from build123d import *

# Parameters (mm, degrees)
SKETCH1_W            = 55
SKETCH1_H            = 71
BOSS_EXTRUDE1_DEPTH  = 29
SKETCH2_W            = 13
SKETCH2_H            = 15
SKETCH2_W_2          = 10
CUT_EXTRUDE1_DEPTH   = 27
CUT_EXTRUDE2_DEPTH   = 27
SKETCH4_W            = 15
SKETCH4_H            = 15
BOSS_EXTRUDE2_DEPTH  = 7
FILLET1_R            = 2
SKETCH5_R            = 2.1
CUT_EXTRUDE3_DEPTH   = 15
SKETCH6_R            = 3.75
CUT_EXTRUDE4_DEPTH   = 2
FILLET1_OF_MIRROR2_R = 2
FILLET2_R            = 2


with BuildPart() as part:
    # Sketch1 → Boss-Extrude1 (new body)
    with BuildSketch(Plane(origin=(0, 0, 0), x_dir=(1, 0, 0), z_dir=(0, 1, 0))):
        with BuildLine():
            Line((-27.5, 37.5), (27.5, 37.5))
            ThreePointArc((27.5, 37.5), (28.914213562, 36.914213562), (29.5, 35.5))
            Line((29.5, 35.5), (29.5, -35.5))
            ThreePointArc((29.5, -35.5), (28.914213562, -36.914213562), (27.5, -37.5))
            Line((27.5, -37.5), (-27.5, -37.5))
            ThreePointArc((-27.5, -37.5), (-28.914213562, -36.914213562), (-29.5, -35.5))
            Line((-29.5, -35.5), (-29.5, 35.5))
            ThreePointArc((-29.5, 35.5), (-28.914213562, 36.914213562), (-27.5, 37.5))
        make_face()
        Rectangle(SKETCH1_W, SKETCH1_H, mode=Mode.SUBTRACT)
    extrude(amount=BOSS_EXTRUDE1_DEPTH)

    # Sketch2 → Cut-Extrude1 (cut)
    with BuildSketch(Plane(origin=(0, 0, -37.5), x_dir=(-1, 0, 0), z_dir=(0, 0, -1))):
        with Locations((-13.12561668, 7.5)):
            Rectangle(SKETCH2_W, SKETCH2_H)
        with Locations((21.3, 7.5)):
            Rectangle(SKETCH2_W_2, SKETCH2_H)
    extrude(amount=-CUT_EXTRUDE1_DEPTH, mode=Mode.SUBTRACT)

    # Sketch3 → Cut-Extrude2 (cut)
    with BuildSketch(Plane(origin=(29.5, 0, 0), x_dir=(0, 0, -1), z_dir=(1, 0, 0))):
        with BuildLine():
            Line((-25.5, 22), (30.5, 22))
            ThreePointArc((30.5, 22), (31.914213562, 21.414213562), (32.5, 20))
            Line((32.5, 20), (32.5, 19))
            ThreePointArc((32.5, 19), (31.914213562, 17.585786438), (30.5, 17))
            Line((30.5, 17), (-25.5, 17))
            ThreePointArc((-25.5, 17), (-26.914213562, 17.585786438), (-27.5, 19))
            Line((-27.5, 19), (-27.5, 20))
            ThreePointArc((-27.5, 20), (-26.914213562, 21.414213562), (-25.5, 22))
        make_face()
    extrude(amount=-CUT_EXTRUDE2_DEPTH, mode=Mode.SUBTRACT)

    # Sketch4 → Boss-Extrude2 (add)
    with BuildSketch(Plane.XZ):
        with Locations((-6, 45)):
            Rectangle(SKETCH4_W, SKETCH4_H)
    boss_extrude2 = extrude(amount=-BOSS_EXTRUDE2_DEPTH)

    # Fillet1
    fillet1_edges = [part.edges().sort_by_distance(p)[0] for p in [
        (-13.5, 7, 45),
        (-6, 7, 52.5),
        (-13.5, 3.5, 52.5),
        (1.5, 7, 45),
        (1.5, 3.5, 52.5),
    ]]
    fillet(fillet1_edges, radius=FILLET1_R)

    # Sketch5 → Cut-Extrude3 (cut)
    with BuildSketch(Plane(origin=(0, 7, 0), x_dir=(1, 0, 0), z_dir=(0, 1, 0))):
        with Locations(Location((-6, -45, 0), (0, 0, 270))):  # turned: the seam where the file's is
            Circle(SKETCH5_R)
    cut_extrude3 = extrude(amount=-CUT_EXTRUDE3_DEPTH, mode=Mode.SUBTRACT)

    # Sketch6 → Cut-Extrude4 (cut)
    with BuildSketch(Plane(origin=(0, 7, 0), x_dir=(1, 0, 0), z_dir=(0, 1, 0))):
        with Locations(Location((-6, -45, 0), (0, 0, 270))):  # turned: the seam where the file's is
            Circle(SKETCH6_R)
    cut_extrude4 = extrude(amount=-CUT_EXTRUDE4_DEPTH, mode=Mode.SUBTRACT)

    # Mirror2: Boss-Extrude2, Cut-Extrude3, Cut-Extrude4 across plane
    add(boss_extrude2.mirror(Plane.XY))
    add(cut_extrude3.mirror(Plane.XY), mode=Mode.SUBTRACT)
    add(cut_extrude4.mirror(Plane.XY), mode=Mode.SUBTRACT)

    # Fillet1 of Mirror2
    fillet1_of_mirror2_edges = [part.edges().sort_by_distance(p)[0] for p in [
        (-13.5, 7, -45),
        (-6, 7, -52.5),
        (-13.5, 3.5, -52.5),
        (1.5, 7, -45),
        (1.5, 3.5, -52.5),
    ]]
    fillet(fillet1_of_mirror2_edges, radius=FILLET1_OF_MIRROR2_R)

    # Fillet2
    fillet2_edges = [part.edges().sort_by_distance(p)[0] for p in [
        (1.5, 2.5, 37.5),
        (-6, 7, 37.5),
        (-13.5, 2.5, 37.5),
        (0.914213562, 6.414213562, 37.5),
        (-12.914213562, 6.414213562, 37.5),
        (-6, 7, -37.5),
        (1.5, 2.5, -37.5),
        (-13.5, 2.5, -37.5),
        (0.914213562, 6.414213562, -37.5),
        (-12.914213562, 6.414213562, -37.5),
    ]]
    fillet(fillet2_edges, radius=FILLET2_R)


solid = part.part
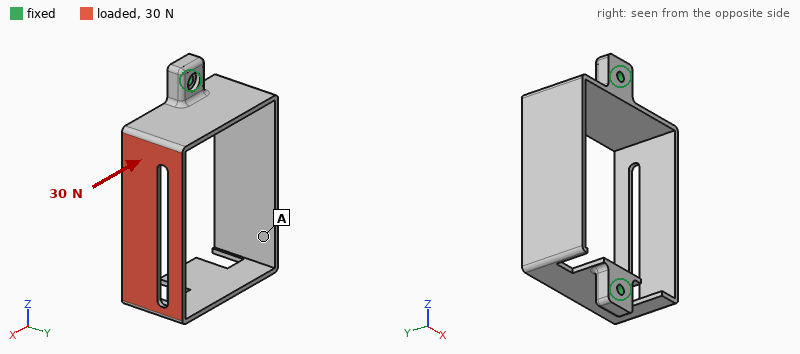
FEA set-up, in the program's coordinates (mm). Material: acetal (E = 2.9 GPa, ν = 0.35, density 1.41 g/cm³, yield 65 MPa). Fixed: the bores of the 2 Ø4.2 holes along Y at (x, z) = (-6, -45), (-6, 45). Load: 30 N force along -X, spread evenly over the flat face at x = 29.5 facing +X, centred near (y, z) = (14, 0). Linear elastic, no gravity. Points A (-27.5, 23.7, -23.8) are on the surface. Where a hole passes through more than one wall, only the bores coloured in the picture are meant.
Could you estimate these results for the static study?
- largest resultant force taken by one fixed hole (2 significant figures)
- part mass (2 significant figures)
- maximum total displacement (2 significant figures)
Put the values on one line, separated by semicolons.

17 N; 23 g; 1.2 mm
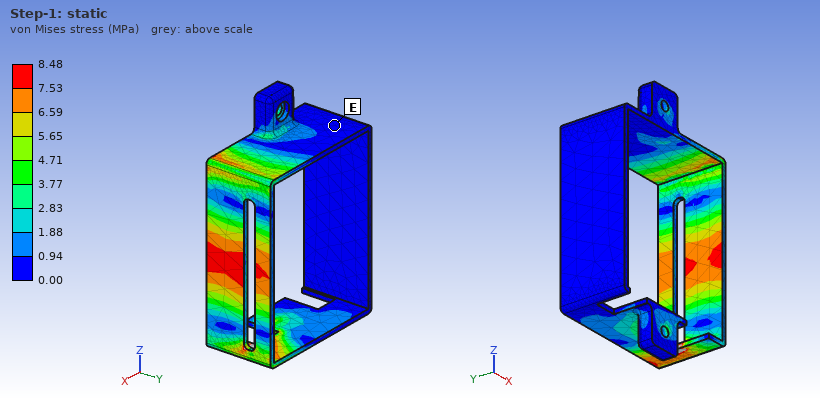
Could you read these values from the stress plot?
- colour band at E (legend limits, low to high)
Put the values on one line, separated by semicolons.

0.00 to 0.94 MPa
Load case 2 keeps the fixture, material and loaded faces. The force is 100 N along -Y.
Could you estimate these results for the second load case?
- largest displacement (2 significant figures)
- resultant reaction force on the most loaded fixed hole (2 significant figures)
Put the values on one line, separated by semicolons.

1.3 mm; 51 N
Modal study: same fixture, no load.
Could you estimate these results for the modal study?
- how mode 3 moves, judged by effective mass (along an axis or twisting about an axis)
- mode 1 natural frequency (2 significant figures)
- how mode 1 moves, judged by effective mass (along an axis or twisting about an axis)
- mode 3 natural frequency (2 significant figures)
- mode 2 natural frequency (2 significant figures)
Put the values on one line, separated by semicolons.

along X; 260 Hz; along Z; 410 Hz; 380 Hz
